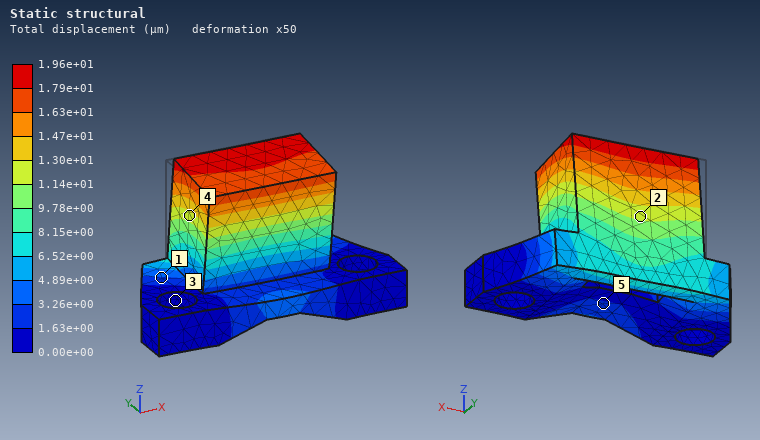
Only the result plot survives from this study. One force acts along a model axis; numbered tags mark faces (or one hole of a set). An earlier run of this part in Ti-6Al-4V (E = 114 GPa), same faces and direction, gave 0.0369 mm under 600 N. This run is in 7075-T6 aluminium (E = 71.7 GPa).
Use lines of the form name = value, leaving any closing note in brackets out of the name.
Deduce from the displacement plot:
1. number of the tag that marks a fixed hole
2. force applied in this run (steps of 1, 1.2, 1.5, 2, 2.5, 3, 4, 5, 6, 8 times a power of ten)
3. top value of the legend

number of the tag that marks a fixed hole = 3
force applied in this run = 200 N
top value of the legend = 1.96e+01 µm
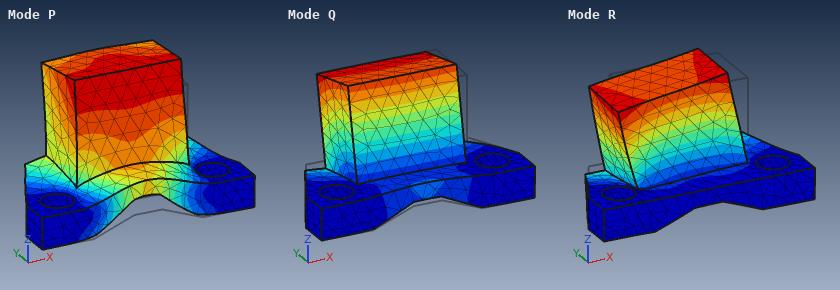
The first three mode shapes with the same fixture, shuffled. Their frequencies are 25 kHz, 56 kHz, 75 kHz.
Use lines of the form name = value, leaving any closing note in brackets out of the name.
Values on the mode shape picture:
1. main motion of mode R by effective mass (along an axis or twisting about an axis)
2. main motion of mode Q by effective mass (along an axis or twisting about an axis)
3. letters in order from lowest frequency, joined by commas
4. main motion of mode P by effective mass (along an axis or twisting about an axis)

main motion of mode R by effective mass = along X
main motion of mode Q by effective mass = along Y
letters in order from lowest frequency, joined by commas = Q, R, P
main motion of mode P by effective mass = along Z
